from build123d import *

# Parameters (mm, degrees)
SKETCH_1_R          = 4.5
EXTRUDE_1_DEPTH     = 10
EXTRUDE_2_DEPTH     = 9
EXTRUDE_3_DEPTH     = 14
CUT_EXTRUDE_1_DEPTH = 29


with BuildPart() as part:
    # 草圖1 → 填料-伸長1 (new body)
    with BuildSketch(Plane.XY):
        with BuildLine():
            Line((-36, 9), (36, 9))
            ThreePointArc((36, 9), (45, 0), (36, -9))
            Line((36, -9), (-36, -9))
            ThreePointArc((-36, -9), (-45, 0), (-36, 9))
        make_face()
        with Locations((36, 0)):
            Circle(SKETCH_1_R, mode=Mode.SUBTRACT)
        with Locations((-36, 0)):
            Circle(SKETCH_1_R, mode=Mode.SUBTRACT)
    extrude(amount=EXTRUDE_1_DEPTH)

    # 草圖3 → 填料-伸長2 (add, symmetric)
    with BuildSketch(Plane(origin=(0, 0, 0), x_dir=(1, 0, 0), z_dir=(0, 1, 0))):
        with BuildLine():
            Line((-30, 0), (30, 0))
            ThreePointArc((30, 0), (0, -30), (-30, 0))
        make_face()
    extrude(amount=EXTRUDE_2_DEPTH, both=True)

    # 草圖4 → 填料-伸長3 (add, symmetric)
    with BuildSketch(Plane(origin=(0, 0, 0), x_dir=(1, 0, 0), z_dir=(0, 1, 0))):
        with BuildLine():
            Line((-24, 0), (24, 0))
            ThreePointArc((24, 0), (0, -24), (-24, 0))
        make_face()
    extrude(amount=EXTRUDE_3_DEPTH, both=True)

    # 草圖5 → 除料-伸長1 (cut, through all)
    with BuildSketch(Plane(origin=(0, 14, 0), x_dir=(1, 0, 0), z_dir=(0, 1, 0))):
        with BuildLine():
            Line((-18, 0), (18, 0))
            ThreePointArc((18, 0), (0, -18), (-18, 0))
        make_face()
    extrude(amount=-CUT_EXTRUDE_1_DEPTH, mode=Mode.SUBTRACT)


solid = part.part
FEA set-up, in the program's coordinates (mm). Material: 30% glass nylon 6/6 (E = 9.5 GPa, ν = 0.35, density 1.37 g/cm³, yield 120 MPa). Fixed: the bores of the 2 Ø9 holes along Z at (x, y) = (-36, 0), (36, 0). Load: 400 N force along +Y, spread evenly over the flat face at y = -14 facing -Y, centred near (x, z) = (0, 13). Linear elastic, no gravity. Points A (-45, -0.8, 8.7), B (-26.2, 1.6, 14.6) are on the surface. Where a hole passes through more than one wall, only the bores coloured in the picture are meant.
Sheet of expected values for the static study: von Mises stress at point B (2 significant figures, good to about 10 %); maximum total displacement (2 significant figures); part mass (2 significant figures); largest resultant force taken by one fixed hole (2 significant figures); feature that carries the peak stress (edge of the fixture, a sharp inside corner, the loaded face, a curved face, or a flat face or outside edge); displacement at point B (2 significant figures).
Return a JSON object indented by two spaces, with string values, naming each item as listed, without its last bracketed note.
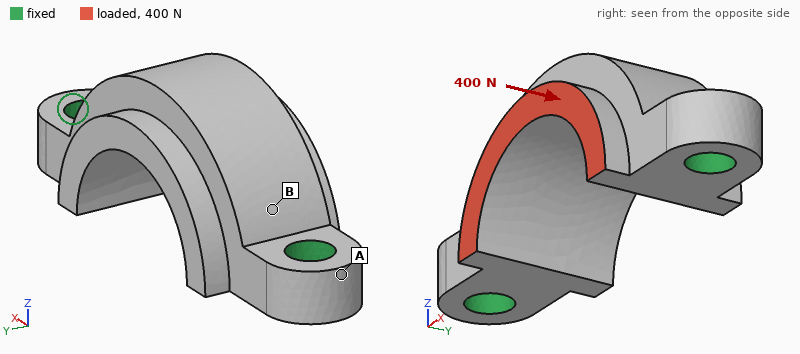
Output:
{
  "von Mises stress at point B": "3.1 MPa",
  "maximum total displacement": "41 µm",
  "part mass": "33 g",
  "largest resultant force taken by one fixed hole": "200 N",
  "feature that carries the peak stress": "edge of the fixture",
  "displacement at point B": "14 µm"
}
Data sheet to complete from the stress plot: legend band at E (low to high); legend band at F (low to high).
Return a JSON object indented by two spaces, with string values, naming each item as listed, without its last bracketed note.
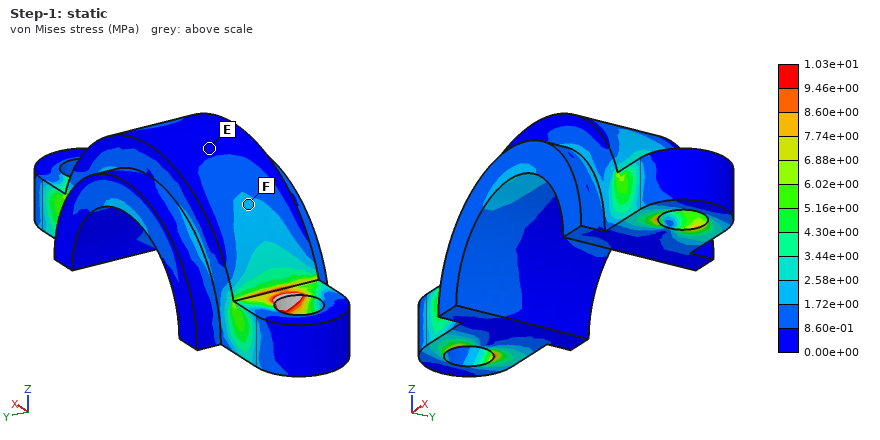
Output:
{
  "legend band at E": "0.00e+00 to 8.60e-01 MPa",
  "legend band at F": "1.72e+00 to 2.58e+00 MPa"
}
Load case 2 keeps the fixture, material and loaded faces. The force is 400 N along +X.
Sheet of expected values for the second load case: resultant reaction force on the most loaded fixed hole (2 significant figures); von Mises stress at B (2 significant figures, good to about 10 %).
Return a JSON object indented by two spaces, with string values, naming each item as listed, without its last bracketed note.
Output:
{
  "resultant reaction force on the most loaded fixed hole": "220 N",
  "von Mises stress at B": "1.2 MPa"
}
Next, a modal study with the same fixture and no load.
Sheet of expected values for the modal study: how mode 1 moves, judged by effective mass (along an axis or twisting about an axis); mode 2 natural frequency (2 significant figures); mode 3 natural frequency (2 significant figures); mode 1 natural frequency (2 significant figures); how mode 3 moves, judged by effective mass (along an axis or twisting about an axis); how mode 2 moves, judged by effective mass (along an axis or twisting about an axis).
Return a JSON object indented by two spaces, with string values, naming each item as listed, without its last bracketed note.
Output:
{
  "how mode 1 moves, judged by effective mass": "along Y",
  "mode 2 natural frequency": "7600 Hz",
  "mode 3 natural frequency": "8500 Hz",
  "mode 1 natural frequency": "3400 Hz",
  "how mode 3 moves, judged by effective mass": "along X",
  "how mode 2 moves, judged by effective mass": "along Z"
}
